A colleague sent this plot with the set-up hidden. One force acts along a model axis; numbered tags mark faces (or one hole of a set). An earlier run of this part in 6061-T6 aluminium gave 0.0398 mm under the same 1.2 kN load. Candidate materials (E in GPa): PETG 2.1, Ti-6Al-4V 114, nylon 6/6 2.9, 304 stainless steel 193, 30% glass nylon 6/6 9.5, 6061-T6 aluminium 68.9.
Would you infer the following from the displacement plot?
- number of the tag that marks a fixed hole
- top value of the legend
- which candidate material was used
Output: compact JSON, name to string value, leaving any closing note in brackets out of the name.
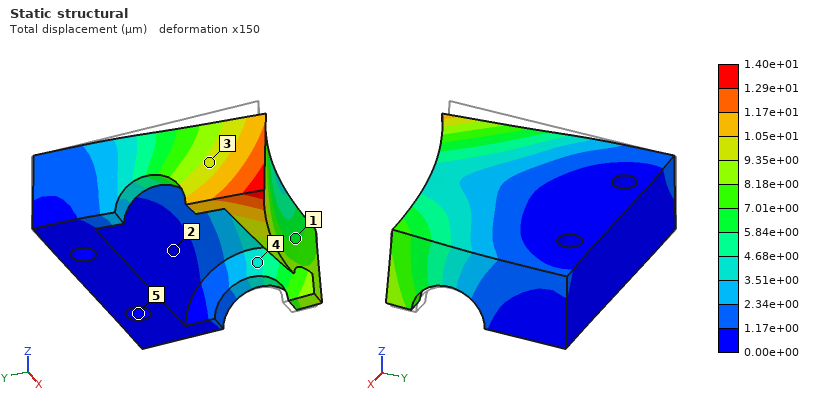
{"number of the tag that marks a fixed hole": "5", "top value of the legend": "1.40e+01 µm", "which candidate material was used": "304 stainless steel"}
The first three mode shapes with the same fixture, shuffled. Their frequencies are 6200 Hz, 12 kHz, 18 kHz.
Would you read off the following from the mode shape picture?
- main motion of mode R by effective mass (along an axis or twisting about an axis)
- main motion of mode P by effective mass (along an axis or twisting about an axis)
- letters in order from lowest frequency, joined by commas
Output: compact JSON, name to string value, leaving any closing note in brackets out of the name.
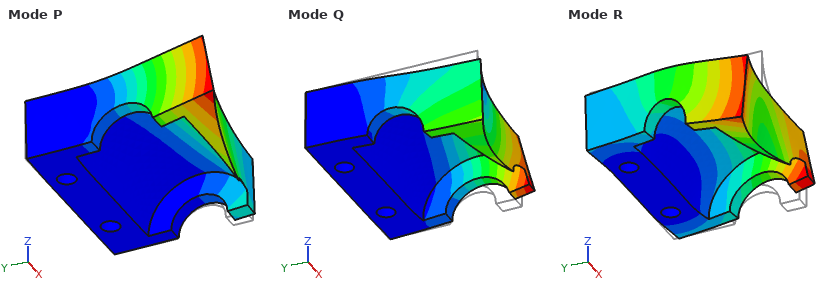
{"main motion of mode R by effective mass": "along X", "main motion of mode P by effective mass": "along Z", "letters in order from lowest frequency, joined by commas": "P, Q, R"}
